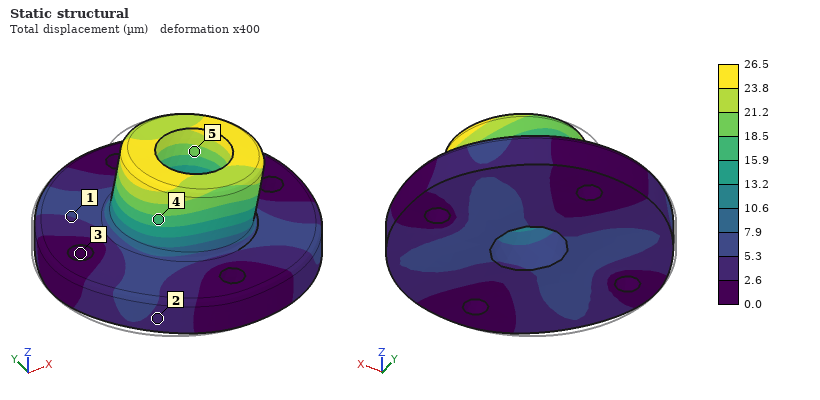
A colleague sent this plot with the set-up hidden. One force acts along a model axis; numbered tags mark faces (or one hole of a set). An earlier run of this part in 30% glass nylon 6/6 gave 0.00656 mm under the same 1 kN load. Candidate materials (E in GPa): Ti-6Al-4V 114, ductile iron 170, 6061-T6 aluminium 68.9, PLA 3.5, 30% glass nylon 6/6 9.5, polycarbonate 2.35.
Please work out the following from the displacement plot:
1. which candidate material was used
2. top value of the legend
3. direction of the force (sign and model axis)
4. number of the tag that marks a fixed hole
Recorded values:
polycarbonate
26.5 µm
+X
3
